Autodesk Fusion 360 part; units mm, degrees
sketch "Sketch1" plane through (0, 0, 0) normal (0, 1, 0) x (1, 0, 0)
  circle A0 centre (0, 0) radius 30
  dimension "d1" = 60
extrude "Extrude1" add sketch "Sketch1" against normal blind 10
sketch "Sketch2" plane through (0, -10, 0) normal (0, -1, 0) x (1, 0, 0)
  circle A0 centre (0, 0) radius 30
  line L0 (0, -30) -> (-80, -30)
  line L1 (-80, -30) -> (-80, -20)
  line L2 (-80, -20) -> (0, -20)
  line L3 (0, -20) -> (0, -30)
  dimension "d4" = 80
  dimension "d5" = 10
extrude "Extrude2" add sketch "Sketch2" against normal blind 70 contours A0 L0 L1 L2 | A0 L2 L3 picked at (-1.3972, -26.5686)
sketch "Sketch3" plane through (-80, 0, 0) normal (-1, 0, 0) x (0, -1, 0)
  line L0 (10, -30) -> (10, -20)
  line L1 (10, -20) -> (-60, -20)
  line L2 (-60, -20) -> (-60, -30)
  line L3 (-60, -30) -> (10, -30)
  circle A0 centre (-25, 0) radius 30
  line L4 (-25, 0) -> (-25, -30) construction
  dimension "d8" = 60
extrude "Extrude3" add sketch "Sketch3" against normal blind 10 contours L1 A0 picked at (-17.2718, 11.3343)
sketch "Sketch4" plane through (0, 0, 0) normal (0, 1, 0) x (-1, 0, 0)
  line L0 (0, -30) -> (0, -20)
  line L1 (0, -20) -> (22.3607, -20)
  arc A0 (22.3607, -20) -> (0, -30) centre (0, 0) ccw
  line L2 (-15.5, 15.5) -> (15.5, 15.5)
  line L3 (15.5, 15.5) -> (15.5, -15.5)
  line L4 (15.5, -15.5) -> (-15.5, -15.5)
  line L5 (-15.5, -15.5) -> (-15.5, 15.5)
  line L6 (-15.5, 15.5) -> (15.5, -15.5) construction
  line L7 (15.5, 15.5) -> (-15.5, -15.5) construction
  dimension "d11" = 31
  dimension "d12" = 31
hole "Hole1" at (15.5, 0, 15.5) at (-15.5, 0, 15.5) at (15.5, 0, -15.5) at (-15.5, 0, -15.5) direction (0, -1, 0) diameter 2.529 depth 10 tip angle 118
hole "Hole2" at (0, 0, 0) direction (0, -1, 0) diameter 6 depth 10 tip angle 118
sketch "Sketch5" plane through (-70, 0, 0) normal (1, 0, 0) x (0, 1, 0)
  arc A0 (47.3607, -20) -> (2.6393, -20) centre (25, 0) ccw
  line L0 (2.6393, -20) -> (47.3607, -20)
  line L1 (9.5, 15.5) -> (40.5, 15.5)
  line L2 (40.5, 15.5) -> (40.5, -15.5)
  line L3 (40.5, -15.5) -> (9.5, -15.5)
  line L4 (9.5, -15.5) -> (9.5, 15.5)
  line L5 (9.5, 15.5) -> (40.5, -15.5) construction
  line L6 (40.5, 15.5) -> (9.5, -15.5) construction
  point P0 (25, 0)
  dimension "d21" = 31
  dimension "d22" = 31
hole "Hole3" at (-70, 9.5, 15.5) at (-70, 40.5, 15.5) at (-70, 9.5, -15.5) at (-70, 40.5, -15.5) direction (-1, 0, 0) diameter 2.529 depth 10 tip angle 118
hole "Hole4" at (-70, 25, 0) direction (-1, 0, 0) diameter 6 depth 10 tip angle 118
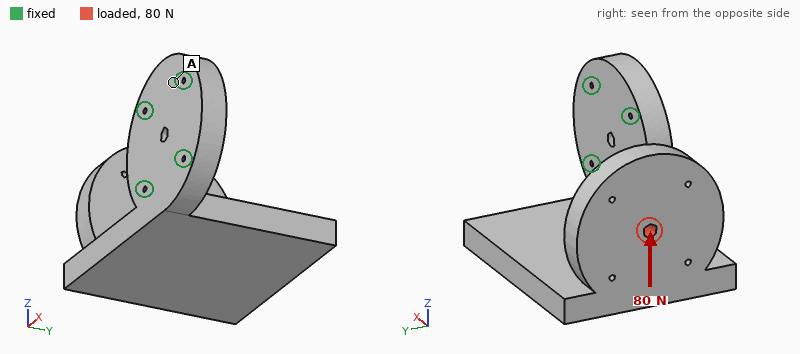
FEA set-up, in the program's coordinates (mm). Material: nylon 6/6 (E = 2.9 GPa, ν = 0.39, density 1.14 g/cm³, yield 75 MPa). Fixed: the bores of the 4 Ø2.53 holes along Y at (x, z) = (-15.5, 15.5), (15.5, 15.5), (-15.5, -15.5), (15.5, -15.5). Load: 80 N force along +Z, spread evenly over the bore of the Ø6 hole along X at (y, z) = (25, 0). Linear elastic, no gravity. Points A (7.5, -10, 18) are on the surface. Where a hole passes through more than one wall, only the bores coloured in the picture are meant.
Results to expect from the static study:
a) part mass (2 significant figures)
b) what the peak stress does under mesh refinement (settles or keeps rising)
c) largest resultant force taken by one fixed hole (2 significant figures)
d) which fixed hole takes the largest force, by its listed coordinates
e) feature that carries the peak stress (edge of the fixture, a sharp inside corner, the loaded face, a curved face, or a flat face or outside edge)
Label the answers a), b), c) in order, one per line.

a) 120 g
b) keeps rising
c) 200 N
d) (-15.5, -15.5)
e) edge of the fixture
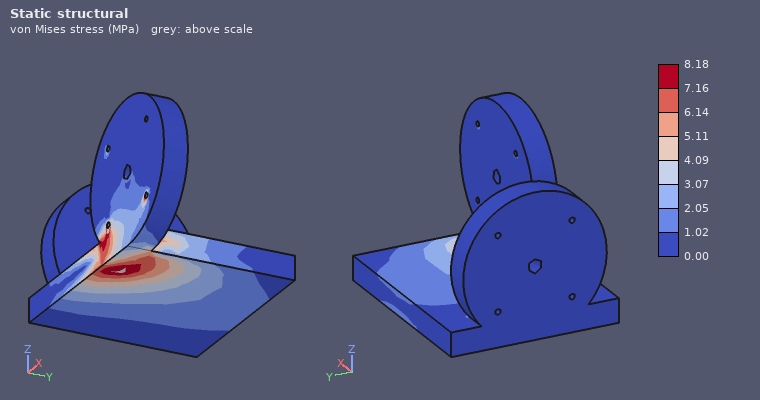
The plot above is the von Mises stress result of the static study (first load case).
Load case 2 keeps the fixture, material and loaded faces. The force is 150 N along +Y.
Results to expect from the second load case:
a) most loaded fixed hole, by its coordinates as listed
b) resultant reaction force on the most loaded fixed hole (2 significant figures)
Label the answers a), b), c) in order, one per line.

a) (-15.5, -15.5)
b) 370 N
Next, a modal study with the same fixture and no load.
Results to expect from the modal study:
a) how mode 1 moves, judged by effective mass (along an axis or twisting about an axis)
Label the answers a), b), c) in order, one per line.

a) along Z
